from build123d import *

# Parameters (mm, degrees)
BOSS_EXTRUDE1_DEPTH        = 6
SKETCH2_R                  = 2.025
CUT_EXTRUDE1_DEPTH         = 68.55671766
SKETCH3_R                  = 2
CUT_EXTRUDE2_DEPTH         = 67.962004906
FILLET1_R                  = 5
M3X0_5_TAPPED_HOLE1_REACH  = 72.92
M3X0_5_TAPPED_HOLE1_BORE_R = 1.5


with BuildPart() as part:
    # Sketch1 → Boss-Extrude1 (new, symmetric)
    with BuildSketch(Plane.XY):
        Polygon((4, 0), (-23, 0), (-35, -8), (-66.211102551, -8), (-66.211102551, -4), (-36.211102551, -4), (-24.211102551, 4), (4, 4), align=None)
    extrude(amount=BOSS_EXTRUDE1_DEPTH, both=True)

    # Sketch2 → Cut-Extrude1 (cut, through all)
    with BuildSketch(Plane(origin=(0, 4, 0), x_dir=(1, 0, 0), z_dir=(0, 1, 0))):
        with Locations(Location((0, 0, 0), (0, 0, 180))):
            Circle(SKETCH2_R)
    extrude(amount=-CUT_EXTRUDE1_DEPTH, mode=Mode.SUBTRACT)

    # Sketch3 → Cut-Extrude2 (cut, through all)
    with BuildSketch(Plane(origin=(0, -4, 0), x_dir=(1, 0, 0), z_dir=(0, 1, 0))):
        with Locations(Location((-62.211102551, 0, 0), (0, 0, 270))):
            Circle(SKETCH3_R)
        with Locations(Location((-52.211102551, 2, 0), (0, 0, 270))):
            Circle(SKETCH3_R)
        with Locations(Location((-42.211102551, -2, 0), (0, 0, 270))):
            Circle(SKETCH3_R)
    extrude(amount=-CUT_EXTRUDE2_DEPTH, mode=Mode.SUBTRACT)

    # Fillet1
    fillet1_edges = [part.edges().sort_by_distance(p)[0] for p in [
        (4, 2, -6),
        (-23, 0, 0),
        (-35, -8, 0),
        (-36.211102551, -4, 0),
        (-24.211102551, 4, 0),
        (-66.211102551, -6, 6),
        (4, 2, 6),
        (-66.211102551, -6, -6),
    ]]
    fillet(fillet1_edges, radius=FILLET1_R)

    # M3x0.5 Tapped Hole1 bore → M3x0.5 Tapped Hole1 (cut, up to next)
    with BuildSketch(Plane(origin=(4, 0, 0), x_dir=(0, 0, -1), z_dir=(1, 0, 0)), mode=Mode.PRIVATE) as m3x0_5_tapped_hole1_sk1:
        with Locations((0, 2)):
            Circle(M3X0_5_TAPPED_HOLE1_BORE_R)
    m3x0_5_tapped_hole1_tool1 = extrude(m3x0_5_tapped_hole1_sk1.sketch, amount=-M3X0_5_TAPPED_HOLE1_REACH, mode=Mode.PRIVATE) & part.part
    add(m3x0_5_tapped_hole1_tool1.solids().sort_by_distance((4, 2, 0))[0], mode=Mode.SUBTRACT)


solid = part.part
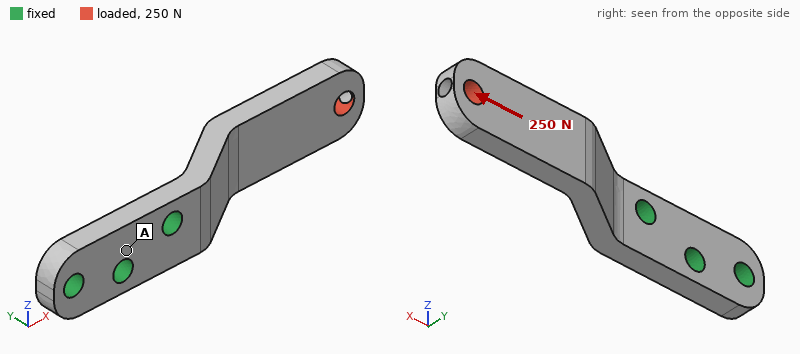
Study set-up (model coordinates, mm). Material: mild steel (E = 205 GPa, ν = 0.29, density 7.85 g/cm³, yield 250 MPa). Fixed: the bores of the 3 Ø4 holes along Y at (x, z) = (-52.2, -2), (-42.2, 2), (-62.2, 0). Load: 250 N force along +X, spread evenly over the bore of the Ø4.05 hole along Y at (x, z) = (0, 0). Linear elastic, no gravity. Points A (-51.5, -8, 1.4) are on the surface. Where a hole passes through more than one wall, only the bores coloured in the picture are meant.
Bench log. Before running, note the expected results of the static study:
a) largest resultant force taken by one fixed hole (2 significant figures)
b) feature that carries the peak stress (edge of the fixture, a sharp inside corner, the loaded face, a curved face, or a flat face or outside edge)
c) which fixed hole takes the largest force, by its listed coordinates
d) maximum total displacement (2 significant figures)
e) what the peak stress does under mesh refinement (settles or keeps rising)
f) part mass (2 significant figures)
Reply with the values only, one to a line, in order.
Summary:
210 N
edge of the fixture
(-42.2, 2)
77 µm
keeps rising
25 g
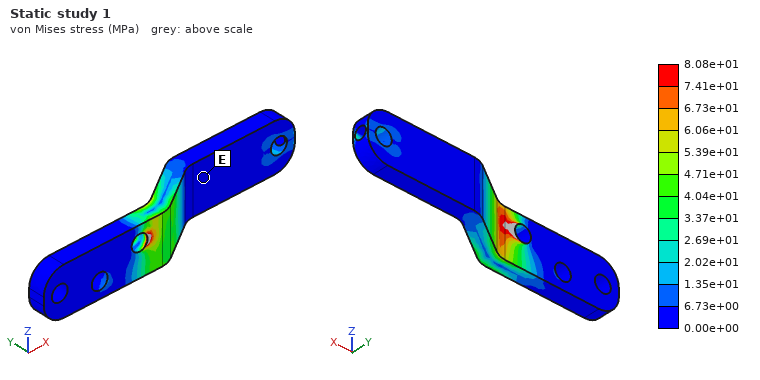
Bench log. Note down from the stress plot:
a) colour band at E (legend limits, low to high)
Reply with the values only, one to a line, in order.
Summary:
0.00e+00 to 6.73e+00 MPa
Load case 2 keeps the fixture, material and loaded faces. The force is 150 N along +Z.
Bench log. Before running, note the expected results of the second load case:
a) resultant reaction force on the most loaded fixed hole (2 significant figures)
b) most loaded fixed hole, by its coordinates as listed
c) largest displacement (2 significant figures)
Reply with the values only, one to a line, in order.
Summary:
490 N
(-42.2, 2)
66 µm
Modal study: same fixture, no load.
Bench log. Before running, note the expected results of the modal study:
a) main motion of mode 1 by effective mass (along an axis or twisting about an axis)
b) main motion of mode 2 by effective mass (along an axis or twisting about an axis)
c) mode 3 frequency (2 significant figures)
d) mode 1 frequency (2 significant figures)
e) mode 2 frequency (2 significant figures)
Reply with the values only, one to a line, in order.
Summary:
along Y
along Z
8700 Hz
1600 Hz
3700 Hz
